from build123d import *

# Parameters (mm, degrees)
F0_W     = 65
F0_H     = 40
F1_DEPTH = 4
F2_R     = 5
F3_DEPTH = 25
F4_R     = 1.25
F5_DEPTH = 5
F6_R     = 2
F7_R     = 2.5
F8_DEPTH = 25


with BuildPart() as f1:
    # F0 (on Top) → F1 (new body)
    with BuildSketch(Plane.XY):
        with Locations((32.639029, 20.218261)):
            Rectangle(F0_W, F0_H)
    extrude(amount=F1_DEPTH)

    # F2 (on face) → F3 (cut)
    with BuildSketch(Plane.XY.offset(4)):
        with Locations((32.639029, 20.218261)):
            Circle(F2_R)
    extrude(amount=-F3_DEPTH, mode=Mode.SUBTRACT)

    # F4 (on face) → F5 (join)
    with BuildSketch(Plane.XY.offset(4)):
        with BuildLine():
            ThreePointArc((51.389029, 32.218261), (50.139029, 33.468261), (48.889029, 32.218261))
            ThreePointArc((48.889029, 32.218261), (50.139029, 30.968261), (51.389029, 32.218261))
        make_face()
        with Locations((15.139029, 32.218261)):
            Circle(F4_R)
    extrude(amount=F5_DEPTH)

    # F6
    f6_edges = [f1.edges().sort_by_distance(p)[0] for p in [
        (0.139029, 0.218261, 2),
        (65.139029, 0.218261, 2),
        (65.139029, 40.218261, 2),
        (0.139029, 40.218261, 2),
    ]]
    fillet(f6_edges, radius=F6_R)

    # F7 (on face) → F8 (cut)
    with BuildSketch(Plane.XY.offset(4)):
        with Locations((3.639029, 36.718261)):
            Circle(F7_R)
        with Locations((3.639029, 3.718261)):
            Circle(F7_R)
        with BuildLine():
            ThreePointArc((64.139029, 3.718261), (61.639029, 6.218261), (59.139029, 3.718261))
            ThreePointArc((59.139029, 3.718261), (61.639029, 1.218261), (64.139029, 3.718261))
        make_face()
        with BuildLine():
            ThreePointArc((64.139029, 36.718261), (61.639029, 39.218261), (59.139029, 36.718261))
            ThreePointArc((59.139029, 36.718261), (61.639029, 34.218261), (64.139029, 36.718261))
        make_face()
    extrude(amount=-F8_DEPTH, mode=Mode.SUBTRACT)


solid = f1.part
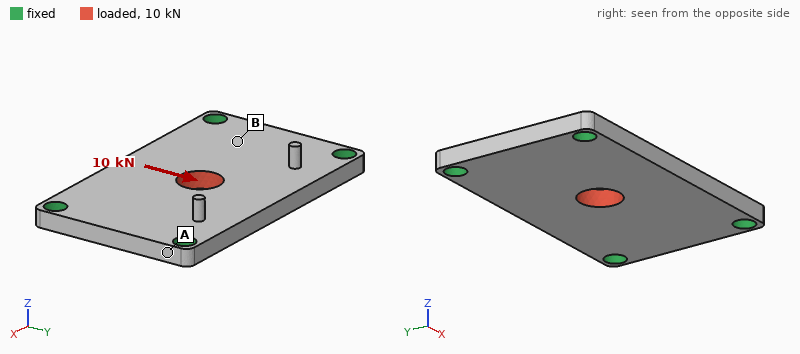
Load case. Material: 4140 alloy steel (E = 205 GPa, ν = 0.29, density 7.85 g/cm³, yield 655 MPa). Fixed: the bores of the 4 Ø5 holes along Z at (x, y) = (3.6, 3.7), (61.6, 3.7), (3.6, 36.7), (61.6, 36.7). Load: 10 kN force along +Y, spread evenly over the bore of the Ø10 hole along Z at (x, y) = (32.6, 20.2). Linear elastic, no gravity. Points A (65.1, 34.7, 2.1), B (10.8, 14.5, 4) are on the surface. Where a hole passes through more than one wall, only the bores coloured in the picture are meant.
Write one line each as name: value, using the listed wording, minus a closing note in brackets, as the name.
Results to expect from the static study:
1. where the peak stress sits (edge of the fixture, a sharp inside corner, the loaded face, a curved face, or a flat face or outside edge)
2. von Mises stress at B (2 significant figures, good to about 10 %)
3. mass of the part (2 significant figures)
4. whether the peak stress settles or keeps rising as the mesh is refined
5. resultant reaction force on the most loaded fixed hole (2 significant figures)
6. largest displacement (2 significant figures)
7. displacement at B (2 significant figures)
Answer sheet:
where the peak stress sits: edge of the fixture
von Mises stress at B: 61 MPa
mass of the part: 77 g
whether the peak stress settles or keeps rising as the mesh is refined: keeps rising
resultant reaction force on the most loaded fixed hole: 3.3 kN
largest displacement: 15 µm
displacement at B: 3.9 µm
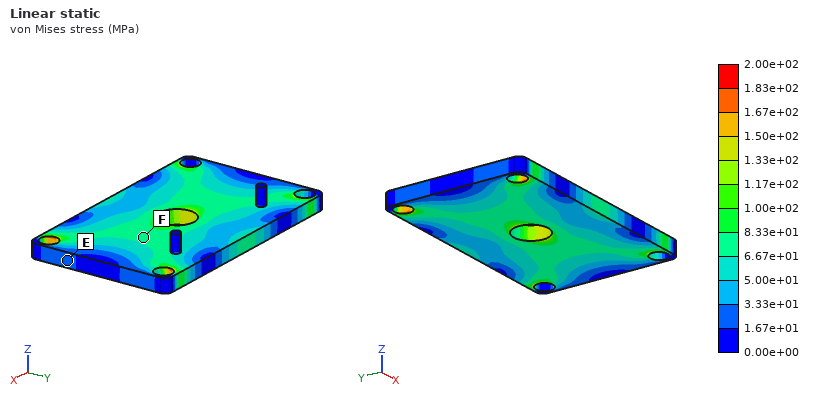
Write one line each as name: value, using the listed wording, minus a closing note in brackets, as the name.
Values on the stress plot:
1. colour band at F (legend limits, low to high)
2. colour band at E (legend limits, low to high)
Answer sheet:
colour band at F: 6.67e+01 to 8.33e+01 MPa
colour band at E: 1.67e+01 to 3.33e+01 MPa
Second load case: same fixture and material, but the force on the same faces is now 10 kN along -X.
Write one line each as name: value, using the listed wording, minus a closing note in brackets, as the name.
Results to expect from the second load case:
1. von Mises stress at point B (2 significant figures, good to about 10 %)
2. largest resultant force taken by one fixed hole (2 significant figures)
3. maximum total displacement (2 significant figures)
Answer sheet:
von Mises stress at point B: 31 MPa
largest resultant force taken by one fixed hole: 2.7 kN
maximum total displacement: 7.9 µm
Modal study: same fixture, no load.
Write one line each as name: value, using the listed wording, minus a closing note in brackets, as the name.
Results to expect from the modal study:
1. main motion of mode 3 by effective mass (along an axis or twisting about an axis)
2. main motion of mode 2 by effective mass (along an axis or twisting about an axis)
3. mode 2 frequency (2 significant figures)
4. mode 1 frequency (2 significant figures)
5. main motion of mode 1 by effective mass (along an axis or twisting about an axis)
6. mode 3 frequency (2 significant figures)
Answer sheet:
main motion of mode 3 by effective mass: twisting about Y
main motion of mode 2 by effective mass: twisting about X
mode 2 frequency: 8900 Hz
mode 1 frequency: 5700 Hz
main motion of mode 1 by effective mass: along Z
mode 3 frequency: 14 kHz
